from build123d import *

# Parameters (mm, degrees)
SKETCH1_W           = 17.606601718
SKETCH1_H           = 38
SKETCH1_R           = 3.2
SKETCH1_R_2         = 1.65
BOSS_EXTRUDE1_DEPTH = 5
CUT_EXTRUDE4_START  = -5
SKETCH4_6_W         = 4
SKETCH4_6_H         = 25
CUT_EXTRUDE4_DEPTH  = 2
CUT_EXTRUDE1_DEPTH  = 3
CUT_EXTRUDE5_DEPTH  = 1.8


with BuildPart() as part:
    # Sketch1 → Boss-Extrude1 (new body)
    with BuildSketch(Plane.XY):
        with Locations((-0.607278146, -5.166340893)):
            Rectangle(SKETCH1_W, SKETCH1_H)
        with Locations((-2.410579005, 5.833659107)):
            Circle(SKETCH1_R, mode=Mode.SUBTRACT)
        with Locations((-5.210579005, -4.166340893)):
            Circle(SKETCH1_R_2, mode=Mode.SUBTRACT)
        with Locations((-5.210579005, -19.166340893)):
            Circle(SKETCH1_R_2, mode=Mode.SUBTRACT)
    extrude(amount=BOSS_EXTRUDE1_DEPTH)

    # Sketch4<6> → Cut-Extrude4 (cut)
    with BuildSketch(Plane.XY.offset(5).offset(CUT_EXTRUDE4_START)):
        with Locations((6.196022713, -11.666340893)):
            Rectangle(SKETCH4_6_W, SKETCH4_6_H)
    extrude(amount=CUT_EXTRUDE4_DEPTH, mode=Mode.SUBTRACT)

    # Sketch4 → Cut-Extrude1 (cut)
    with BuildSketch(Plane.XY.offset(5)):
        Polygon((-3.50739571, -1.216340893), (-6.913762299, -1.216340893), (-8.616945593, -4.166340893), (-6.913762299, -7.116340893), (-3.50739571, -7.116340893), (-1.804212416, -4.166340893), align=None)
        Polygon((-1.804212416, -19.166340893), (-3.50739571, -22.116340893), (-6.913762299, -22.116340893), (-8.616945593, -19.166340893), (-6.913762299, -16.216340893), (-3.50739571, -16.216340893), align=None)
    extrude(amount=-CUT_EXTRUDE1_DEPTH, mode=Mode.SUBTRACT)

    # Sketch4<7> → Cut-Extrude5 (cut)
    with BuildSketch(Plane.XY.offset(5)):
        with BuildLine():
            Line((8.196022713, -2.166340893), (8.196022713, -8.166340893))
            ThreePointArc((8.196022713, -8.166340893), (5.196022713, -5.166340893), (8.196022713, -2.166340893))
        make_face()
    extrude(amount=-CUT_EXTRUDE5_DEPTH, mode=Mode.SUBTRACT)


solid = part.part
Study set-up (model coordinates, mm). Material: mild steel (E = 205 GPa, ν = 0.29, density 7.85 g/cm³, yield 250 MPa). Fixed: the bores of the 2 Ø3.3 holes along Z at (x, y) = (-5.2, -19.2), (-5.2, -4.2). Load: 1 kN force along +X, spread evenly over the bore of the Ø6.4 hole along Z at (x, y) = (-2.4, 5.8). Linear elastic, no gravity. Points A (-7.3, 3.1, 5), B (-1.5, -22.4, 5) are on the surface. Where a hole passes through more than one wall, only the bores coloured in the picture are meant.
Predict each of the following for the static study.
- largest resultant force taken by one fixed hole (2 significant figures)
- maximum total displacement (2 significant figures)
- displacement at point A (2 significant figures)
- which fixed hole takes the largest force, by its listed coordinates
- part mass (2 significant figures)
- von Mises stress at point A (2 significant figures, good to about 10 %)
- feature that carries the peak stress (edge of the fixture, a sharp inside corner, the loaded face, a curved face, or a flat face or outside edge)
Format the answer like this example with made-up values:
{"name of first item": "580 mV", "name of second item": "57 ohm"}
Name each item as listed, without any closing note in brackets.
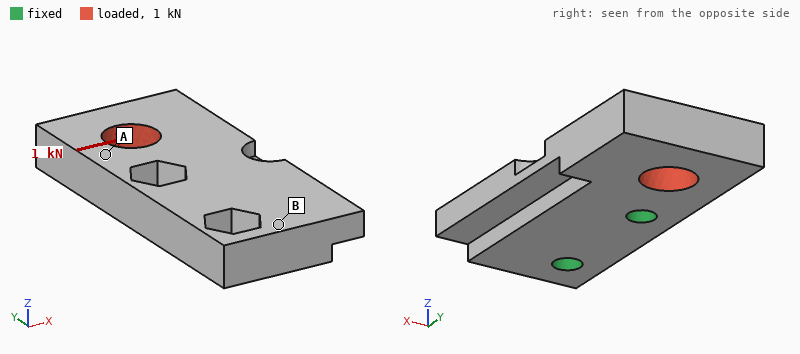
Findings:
{"largest resultant force taken by one fixed hole": "1.5 kN", "maximum total displacement": "21 µm", "displacement at point A": "8.1 µm", "which fixed hole takes the largest force, by its listed coordinates": "(-5.2, -4.2)", "part mass": "22 g", "von Mises stress at point A": "36 MPa", "feature that carries the peak stress": "edge of the fixture"}
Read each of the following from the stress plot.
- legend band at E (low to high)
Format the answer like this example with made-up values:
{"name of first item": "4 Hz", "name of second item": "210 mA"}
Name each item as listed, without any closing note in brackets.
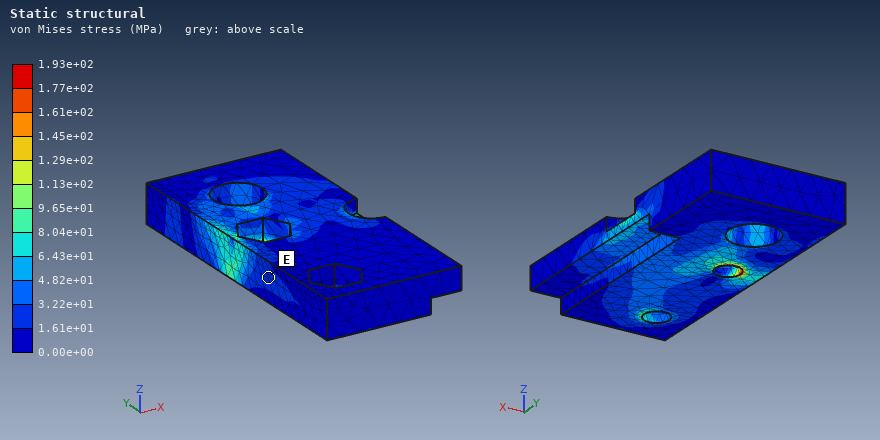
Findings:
{"legend band at E": "1.61e+01 to 3.22e+01 MPa"}
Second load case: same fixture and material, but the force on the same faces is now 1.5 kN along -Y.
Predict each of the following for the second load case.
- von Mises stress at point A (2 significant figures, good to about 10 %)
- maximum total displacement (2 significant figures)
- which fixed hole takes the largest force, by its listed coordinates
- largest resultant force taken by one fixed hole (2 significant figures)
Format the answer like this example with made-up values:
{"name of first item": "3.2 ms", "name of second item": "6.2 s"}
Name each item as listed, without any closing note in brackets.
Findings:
{"von Mises stress at point A": "21 MPa", "maximum total displacement": "7.7 µm", "which fixed hole takes the largest force, by its listed coordinates": "(-5.2, -4.2)", "largest resultant force taken by one fixed hole": "1.1 kN"}
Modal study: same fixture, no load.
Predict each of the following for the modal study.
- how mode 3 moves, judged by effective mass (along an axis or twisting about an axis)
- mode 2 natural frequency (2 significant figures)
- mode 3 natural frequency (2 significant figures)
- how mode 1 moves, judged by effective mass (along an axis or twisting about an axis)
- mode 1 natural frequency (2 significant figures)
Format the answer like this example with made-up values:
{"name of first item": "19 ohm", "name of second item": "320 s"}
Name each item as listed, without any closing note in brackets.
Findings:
{"how mode 3 moves, judged by effective mass": "along X", "mode 2 natural frequency": "11 kHz", "mode 3 natural frequency": "16 kHz", "how mode 1 moves, judged by effective mass": "along Z", "mode 1 natural frequency": "6900 Hz"}
